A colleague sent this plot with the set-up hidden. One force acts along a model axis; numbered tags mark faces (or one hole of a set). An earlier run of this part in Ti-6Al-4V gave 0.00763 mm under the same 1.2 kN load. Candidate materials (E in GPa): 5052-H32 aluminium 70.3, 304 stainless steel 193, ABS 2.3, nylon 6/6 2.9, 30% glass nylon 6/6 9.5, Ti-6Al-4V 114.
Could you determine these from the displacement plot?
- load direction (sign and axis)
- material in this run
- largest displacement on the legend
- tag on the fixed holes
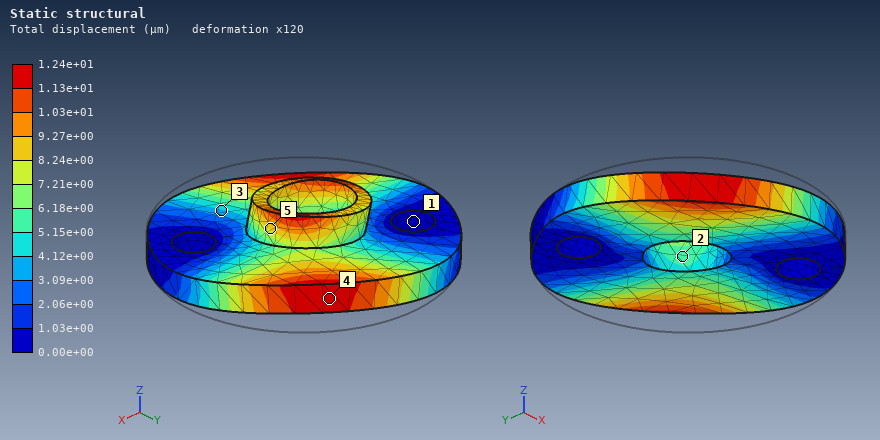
-X
5052-H32 aluminium
1.24e+01 µm
1
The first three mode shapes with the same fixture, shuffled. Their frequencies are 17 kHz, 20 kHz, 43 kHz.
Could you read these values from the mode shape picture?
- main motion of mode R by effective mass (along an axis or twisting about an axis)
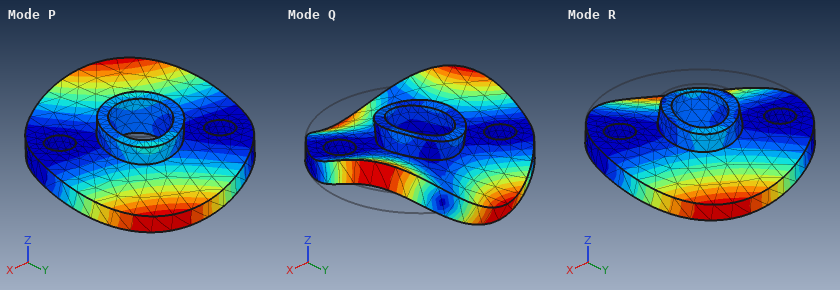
along Z
